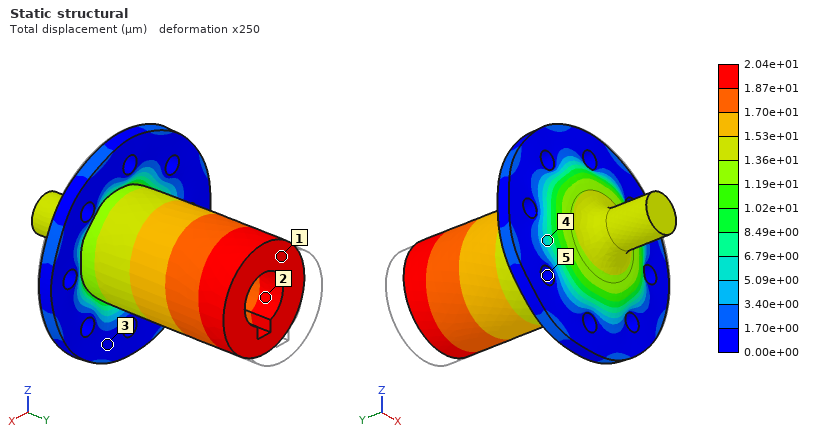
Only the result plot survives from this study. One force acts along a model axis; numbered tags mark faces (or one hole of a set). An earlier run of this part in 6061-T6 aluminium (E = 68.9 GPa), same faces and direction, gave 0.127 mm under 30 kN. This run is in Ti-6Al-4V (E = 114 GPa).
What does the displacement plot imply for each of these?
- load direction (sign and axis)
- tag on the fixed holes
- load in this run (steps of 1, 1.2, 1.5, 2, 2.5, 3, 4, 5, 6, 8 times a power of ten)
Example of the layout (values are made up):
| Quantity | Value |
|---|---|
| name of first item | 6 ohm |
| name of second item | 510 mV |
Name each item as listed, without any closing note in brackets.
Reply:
| Quantity | Value |
|---|---|
| load direction | -Y |
| tag on the fixed holes | 5 |
| load in this run | 8 kN |
